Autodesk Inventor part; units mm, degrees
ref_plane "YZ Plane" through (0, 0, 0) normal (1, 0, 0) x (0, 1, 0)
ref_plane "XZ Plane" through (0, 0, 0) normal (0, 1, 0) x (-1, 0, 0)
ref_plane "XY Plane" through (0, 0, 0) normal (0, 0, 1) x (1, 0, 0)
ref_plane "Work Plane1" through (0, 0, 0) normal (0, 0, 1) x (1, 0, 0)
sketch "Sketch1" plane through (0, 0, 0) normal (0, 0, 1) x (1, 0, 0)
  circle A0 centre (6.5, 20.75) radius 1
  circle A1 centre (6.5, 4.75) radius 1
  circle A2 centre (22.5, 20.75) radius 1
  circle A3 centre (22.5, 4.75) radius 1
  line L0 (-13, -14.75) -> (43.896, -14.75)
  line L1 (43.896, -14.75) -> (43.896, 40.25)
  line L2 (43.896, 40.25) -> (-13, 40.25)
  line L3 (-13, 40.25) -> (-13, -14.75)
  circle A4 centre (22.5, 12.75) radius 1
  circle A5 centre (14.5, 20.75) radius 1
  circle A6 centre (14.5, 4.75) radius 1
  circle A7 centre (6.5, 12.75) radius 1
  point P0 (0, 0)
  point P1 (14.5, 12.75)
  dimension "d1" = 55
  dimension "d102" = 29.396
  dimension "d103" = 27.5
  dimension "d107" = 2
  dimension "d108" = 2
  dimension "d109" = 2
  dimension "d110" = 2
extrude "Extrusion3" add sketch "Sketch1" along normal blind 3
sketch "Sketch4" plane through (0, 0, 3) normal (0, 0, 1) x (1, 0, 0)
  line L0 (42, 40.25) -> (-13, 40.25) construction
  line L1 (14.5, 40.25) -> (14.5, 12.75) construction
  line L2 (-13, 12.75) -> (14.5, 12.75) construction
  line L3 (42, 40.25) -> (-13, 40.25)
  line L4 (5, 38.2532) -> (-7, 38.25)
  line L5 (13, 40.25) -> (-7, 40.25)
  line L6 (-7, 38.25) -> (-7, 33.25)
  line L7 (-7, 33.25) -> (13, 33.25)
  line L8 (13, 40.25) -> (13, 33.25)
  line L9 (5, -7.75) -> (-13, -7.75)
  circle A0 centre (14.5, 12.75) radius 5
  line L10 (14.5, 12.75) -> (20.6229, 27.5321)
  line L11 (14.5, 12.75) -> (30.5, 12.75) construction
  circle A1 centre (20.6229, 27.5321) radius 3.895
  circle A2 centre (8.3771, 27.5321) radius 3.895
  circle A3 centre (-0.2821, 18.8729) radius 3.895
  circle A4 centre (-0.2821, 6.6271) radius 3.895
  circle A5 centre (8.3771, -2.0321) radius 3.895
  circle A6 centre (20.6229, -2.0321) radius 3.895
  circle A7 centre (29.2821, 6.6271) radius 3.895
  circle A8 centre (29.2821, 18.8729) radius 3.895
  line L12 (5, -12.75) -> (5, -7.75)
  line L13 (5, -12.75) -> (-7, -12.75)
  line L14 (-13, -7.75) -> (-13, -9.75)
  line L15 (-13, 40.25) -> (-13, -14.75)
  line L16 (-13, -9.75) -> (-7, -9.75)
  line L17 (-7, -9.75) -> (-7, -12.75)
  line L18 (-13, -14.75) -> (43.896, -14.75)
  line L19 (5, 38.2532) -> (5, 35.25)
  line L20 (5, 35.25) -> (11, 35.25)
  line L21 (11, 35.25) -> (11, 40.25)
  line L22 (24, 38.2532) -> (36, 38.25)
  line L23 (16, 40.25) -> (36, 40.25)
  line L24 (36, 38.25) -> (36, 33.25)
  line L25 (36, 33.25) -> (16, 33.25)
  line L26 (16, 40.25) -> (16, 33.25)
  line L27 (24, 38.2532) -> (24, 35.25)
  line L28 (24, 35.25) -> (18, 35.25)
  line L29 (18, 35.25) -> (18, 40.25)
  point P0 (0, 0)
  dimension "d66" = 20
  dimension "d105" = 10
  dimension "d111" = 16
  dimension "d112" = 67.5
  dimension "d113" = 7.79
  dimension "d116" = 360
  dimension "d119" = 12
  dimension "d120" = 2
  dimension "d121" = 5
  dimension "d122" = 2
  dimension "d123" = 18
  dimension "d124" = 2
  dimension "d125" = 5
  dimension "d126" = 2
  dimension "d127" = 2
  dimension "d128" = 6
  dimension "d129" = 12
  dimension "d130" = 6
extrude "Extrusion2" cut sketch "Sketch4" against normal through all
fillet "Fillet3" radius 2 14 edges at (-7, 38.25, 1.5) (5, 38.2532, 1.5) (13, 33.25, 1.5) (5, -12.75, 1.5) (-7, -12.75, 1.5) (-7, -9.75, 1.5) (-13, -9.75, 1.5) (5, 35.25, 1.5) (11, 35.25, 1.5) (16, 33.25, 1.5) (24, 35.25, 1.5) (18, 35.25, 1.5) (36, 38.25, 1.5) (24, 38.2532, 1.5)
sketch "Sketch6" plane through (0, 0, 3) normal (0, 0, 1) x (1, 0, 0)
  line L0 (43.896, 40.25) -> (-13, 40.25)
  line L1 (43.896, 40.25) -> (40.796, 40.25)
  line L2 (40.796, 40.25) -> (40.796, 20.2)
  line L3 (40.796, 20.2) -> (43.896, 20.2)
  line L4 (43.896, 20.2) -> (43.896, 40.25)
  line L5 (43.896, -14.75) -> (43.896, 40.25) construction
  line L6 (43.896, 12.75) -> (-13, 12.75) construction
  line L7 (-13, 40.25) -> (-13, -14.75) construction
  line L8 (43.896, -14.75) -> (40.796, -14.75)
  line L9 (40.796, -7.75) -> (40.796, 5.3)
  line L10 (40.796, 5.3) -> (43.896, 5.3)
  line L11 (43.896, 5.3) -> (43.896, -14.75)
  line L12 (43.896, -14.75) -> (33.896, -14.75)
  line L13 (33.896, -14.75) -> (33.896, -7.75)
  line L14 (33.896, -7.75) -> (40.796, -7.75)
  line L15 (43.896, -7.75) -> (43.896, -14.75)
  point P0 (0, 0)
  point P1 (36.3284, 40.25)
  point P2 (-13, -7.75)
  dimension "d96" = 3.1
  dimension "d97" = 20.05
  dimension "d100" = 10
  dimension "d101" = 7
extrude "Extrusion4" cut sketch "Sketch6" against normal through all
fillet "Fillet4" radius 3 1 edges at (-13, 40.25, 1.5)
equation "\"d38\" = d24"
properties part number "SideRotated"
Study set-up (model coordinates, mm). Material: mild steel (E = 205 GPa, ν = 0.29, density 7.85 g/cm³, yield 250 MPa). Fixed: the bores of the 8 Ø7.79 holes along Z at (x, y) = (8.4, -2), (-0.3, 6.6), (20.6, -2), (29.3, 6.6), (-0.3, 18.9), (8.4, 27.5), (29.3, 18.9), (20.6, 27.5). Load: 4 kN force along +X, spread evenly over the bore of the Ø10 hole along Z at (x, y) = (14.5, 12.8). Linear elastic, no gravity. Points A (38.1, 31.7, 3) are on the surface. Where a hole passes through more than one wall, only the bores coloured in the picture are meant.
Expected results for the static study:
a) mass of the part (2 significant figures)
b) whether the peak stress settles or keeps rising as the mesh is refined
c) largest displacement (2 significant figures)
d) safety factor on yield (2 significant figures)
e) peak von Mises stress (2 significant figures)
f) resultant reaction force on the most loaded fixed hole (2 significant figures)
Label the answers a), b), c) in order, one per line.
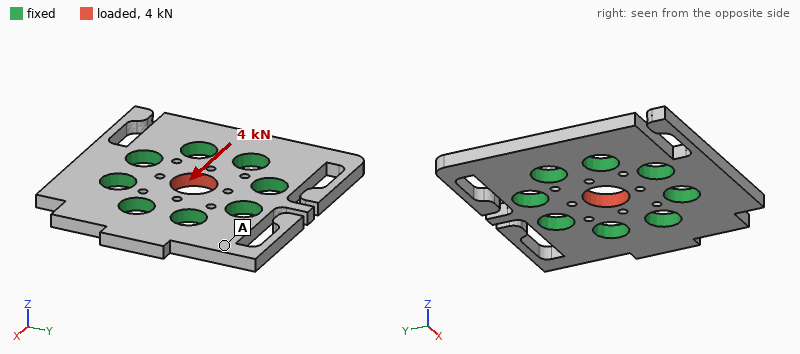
a) 52 g
b) settles
c) 1.8 µm
d) 2.2
e) 110 MPa
f) 830 N
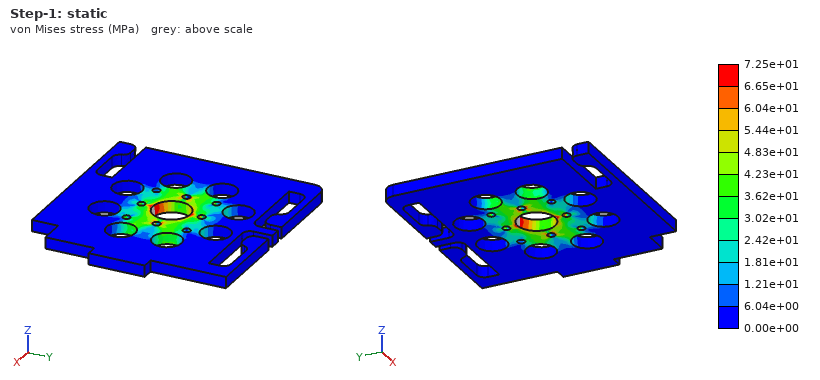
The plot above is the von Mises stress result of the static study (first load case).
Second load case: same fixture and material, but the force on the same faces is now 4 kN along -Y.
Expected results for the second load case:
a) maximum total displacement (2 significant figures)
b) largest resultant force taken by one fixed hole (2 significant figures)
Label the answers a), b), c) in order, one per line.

a) 1.8 µm
b) 830 N
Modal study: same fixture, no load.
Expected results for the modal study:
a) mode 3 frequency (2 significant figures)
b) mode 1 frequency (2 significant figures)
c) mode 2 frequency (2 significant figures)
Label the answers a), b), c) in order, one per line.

a) 3300 Hz
b) 3200 Hz
c) 3300 Hz
